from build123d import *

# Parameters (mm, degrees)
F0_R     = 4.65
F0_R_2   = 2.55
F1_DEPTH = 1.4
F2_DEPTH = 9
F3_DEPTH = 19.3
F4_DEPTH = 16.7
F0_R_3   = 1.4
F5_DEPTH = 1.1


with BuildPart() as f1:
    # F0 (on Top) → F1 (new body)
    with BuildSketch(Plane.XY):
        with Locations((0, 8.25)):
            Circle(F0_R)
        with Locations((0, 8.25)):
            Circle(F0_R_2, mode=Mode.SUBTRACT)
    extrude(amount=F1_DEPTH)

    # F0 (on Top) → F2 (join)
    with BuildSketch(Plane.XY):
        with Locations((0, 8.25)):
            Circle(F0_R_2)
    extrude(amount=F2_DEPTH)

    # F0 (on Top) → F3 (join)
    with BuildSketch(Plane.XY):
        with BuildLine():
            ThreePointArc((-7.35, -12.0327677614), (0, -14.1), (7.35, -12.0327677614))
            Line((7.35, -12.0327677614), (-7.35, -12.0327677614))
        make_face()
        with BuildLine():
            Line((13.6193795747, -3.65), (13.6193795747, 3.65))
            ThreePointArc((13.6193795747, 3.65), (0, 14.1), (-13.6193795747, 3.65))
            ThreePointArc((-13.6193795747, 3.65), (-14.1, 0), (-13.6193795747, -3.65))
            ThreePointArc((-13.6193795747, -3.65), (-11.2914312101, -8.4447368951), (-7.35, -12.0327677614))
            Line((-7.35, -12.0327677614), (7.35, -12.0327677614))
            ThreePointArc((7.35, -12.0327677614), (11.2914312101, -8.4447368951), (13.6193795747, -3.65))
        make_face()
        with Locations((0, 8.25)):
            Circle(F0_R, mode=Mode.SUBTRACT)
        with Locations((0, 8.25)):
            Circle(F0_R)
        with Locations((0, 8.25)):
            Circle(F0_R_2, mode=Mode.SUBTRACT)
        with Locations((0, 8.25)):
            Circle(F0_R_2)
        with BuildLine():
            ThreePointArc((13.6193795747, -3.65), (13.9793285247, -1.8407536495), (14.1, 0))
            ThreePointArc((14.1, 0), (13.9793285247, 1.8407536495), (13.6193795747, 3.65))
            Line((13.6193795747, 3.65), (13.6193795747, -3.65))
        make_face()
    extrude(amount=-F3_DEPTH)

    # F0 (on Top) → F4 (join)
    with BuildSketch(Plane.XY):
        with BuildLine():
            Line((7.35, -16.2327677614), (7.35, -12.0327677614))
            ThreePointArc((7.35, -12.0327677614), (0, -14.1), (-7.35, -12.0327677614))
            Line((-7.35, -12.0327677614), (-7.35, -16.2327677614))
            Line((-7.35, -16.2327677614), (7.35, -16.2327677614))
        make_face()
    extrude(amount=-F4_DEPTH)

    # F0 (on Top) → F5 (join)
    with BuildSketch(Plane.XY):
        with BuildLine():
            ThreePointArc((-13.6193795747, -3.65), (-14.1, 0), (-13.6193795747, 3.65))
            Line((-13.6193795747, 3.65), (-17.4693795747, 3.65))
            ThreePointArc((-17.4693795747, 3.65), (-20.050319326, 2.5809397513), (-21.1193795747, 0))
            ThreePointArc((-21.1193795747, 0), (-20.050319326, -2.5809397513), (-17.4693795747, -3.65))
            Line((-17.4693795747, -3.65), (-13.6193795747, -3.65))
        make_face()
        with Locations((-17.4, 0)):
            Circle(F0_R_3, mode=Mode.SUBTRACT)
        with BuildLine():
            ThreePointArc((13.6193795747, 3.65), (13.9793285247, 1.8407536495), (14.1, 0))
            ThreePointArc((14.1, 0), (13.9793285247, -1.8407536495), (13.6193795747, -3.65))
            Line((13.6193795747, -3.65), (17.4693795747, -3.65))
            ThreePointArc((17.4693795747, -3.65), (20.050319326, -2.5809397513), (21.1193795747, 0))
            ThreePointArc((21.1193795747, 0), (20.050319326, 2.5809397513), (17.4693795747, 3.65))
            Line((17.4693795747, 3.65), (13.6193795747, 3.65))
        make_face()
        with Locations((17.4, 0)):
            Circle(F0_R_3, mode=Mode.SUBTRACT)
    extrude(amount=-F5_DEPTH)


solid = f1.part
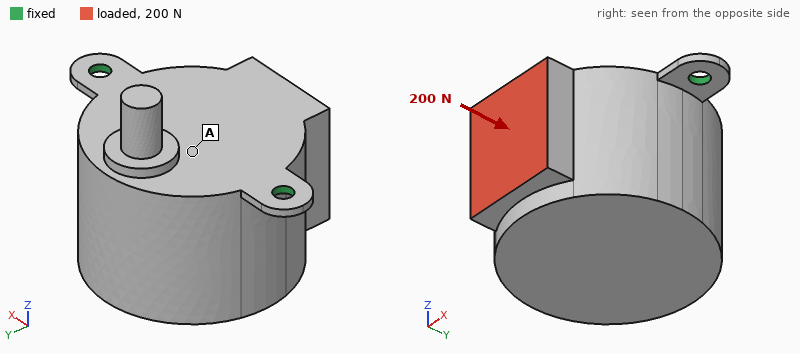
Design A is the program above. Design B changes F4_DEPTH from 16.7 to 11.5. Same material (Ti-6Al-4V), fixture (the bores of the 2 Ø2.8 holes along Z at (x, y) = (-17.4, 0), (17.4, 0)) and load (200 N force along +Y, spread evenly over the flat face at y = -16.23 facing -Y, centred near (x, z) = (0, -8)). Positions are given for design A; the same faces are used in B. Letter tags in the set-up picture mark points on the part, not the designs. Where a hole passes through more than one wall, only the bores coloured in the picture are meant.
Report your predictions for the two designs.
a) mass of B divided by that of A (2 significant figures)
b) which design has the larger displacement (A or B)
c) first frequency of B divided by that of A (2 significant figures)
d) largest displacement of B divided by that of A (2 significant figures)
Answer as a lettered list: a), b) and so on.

a) 0.98
b) A
c) 1.0
d) 0.67
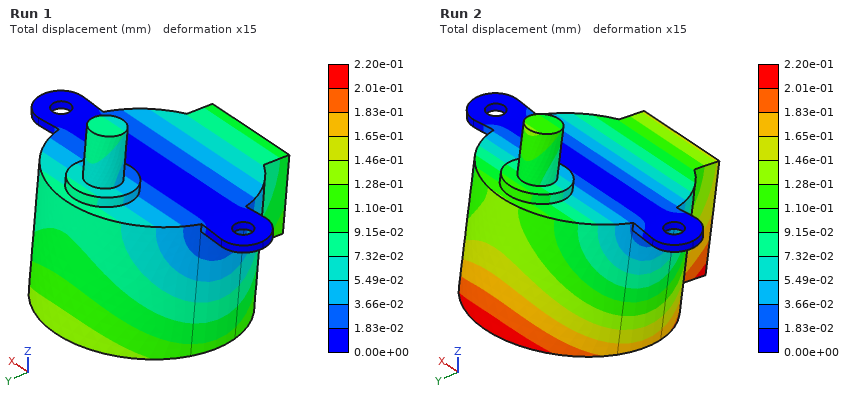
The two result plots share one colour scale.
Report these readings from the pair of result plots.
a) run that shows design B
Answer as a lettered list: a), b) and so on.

a) Run 1
